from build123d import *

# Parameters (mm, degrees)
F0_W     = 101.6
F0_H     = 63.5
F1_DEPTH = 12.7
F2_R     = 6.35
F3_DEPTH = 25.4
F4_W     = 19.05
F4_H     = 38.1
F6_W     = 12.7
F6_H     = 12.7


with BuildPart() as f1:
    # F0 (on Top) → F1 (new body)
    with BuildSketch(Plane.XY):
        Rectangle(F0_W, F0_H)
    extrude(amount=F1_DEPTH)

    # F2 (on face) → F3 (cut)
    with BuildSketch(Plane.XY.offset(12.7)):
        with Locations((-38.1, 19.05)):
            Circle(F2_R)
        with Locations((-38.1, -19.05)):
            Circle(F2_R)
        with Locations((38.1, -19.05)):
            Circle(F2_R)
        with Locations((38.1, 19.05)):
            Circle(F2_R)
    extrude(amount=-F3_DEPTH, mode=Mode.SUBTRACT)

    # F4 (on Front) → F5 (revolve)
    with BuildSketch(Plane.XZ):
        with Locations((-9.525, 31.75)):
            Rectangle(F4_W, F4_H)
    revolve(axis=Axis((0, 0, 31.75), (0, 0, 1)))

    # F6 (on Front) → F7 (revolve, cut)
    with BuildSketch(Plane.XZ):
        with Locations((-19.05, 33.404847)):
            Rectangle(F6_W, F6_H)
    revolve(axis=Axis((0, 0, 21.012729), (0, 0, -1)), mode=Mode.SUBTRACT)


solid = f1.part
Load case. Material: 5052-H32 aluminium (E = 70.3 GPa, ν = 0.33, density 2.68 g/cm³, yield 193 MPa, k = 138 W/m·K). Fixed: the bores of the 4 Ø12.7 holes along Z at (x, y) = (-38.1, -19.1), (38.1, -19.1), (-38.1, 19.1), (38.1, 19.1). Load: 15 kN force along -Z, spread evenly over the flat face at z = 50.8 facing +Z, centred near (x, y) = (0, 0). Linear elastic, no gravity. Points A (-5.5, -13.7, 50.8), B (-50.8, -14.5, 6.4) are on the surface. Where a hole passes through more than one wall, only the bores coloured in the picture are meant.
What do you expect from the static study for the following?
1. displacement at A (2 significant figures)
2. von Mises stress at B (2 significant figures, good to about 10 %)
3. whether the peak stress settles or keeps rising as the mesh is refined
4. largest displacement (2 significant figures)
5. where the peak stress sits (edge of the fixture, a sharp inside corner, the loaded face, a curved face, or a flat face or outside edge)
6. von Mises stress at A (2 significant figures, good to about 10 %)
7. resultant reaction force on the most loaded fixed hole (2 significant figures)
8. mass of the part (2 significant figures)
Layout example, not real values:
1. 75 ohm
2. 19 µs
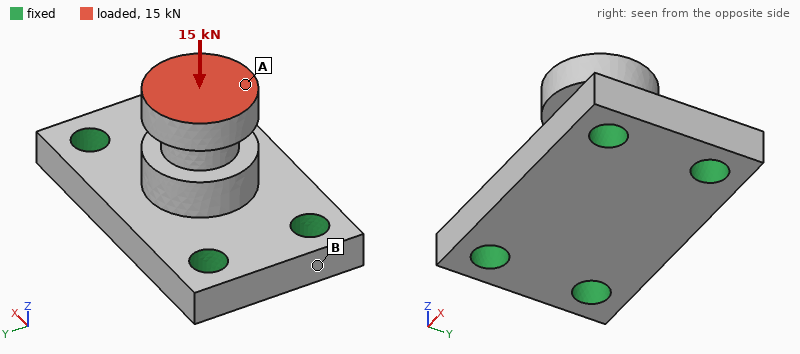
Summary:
1. 40 µm
2. 7.9 MPa
3. keeps rising
4. 41 µm
5. edge of the fixture
6. 20 MPa
7. 3.9 kN
8. 300 g
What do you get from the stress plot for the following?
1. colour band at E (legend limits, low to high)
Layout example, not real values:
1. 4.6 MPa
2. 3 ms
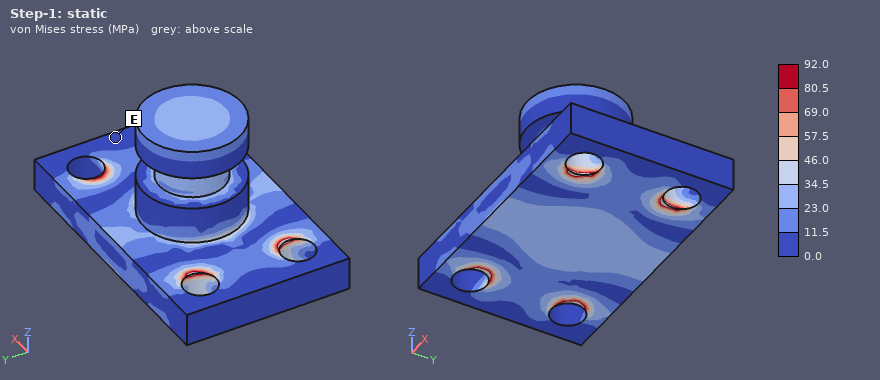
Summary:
1. 0.0 to 11.5 MPa
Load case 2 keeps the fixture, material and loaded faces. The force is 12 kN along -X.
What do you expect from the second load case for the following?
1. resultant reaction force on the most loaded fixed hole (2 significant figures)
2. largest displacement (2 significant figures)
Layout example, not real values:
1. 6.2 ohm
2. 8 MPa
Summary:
1. 5.9 kN
2. 0.19 mm
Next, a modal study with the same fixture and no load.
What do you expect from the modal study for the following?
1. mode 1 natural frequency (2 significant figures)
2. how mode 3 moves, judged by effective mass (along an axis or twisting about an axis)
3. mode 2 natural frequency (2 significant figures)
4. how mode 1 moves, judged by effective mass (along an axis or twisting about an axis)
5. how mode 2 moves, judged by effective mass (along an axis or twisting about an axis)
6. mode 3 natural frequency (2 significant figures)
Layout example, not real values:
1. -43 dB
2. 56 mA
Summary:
1. 5900 Hz
2. along Z
3. 7500 Hz
4. along Y
5. along X
6. 8900 Hz
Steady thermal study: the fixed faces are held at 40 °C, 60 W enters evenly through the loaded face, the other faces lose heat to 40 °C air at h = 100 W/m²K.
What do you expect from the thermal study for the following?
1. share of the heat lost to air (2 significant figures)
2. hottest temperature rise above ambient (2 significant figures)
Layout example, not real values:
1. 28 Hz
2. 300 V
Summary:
1. 20 %
2. 29 K
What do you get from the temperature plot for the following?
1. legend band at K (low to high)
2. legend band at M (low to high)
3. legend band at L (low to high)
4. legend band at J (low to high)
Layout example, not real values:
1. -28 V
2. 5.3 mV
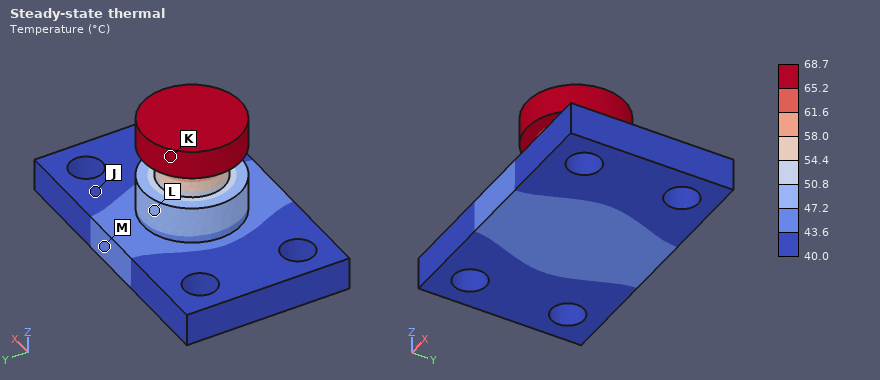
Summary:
1. 65.2 to 68.7 °C
2. 43.6 to 47.2 °C
3. 47.2 to 50.8 °C
4. 40.0 to 43.6 °C
